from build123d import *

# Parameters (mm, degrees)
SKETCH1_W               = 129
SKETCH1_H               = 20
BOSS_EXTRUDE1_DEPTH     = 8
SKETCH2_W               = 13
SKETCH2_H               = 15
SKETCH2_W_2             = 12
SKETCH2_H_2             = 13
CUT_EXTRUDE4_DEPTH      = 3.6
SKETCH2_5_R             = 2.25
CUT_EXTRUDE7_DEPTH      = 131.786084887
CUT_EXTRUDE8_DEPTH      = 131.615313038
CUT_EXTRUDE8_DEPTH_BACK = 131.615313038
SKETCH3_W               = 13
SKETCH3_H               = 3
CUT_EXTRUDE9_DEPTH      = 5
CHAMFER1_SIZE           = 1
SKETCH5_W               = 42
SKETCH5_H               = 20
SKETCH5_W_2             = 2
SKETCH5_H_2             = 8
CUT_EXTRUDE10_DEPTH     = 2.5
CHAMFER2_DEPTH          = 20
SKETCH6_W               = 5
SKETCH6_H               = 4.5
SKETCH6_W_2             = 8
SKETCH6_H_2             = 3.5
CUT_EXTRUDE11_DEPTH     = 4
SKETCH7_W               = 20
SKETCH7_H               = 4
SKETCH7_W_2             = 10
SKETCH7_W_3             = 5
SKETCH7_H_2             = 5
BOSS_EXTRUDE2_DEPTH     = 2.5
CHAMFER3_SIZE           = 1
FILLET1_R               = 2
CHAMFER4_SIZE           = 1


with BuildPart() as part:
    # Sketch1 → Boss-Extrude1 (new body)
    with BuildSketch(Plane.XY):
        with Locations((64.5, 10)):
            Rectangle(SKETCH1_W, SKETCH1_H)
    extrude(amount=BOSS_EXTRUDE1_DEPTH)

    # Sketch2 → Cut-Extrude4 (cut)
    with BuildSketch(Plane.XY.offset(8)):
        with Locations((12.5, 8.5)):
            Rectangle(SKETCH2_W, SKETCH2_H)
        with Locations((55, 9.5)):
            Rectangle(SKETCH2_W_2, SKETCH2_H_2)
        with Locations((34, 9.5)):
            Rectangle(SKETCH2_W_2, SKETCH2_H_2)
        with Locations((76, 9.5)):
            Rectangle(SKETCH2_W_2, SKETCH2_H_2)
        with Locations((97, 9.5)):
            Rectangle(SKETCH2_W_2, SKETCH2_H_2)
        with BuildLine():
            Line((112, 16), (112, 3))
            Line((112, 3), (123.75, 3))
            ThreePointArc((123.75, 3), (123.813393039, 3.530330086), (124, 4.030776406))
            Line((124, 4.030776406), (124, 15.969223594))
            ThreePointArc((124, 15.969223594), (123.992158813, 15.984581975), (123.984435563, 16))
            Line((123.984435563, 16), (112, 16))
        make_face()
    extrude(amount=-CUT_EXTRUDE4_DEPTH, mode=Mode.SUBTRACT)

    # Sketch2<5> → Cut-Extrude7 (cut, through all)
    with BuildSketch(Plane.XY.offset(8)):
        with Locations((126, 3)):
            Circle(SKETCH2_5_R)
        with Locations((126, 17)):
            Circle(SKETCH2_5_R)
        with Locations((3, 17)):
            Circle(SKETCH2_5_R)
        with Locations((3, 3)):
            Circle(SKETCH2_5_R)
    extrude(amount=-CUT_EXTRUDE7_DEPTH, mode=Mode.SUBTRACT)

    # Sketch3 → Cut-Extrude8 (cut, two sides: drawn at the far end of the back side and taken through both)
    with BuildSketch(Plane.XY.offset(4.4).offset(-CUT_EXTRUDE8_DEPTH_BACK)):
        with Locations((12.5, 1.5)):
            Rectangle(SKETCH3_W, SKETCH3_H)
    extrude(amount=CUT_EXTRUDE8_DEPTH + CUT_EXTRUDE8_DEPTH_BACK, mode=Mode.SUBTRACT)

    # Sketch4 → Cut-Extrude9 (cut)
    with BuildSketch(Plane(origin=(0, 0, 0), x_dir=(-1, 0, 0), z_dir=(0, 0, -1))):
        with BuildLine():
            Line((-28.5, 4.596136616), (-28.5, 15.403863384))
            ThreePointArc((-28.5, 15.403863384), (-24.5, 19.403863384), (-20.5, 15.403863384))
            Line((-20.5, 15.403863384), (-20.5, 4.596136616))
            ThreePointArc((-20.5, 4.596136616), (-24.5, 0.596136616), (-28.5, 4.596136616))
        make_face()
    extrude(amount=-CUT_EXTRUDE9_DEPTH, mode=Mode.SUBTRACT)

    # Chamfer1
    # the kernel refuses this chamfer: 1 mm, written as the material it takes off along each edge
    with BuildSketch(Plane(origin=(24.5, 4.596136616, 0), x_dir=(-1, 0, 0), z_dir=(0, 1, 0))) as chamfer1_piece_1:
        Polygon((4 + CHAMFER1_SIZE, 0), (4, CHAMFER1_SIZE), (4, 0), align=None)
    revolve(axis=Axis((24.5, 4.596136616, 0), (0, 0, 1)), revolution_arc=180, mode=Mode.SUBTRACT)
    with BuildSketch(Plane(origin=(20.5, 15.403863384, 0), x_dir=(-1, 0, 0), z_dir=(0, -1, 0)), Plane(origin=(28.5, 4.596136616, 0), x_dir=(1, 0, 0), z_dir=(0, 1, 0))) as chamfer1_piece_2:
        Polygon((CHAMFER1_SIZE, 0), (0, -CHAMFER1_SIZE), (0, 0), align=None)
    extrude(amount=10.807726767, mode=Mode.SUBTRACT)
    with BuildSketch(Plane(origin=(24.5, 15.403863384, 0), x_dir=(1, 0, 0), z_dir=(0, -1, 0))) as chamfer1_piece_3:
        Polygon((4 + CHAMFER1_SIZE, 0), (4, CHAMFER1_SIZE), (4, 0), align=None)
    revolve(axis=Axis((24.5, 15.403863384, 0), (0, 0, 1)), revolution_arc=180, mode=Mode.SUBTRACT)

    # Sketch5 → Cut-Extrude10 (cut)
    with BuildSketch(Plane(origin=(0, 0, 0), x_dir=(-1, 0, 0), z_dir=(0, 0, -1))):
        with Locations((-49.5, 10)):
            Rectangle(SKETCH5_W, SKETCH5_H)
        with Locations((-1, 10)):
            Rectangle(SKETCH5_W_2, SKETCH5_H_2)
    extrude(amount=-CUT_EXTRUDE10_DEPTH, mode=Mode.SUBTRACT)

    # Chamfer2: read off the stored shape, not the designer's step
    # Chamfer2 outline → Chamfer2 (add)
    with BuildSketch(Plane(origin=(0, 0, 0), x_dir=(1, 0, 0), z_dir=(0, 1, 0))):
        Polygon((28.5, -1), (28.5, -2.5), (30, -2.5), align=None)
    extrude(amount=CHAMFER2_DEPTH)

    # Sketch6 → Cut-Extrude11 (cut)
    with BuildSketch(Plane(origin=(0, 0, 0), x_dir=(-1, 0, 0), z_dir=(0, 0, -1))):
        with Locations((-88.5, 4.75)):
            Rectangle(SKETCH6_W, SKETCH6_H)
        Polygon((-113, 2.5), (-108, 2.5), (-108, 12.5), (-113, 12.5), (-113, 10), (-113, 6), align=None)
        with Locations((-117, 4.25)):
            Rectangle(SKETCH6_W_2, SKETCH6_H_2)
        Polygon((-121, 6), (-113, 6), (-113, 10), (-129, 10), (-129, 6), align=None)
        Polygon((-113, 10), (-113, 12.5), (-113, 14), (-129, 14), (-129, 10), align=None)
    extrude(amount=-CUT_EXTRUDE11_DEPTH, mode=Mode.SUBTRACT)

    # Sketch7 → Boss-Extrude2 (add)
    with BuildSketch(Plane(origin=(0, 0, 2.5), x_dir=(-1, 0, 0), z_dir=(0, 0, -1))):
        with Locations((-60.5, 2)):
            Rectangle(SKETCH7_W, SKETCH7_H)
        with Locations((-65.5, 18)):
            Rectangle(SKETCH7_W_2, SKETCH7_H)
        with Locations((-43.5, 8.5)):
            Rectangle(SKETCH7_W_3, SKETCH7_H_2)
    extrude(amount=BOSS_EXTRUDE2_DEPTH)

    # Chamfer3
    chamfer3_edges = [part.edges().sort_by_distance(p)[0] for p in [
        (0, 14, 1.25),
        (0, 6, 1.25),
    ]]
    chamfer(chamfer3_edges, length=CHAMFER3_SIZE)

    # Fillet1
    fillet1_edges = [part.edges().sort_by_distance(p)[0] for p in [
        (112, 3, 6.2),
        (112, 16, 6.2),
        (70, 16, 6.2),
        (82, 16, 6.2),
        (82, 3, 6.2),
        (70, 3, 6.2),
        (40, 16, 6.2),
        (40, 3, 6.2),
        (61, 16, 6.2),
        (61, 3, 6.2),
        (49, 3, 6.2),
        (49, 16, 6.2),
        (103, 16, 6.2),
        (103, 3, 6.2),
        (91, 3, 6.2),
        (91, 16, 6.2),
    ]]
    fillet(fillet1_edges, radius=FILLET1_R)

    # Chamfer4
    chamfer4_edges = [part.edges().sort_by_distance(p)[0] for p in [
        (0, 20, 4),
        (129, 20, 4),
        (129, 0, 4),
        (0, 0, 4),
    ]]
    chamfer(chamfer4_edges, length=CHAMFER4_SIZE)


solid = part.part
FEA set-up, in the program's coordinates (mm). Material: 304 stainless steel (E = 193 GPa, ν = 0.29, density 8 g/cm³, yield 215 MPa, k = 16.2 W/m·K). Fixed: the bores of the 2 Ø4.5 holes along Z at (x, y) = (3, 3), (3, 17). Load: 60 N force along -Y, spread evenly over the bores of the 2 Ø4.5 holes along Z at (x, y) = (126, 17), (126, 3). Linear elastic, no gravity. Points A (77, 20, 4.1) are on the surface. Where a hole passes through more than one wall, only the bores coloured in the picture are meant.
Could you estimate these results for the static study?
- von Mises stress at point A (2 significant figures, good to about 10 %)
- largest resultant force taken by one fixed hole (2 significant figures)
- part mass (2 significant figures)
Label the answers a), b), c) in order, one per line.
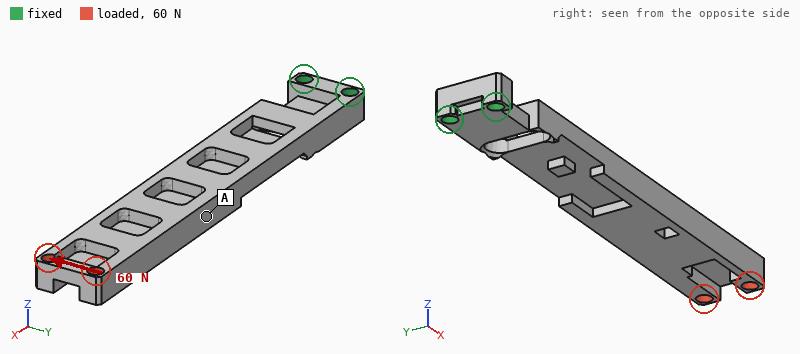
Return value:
a) 6.1 MPa
b) 530 N
c) 100 g
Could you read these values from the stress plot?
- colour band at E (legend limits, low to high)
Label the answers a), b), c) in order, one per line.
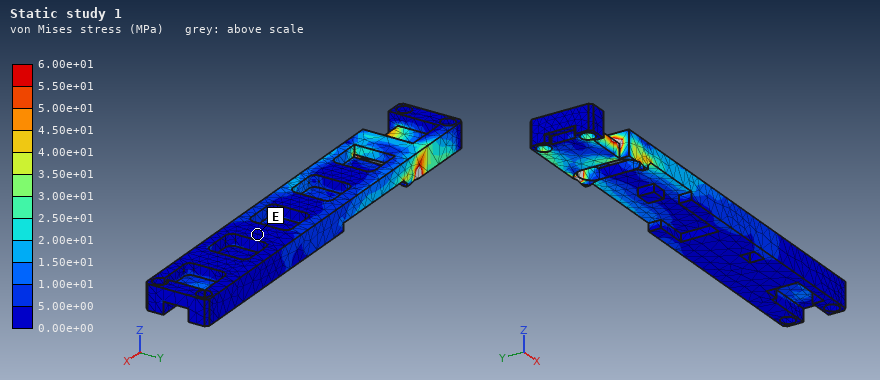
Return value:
a) 0.00e+00 to 5.00e+00 MPa
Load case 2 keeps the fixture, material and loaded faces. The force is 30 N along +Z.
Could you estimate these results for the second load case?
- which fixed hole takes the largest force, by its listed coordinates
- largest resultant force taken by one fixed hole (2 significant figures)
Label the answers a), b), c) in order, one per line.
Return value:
a) (3, 17)
b) 44 N
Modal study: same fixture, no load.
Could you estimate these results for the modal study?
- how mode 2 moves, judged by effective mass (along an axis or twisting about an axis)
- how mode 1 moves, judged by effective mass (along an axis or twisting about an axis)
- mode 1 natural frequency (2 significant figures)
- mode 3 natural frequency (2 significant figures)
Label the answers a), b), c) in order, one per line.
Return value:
a) along Y
b) along Z
c) 210 Hz
d) 1800 Hz
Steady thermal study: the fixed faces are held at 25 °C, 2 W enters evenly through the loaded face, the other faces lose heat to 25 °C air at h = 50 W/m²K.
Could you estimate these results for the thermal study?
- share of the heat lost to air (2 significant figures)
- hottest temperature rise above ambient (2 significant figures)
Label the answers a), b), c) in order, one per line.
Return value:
a) 100 %
b) 29 K
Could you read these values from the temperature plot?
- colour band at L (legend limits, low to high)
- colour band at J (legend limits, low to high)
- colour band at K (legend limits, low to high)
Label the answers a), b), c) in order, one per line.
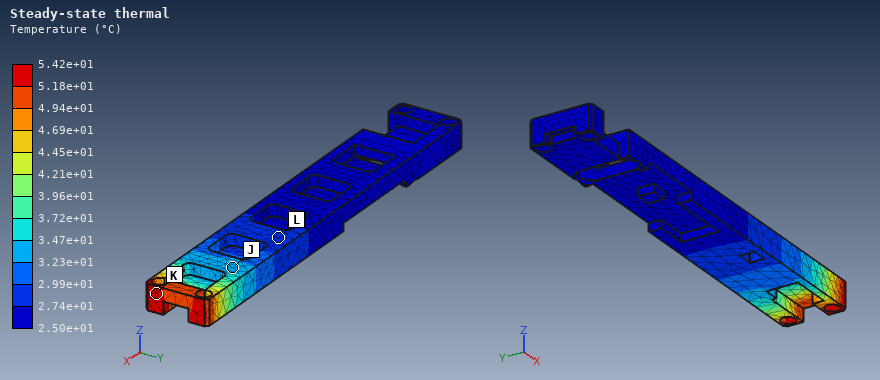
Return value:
a) 2.74e+01 to 2.99e+01 °C
b) 3.23e+01 to 3.47e+01 °C
c) 5.18e+01 to 5.42e+01 °C
